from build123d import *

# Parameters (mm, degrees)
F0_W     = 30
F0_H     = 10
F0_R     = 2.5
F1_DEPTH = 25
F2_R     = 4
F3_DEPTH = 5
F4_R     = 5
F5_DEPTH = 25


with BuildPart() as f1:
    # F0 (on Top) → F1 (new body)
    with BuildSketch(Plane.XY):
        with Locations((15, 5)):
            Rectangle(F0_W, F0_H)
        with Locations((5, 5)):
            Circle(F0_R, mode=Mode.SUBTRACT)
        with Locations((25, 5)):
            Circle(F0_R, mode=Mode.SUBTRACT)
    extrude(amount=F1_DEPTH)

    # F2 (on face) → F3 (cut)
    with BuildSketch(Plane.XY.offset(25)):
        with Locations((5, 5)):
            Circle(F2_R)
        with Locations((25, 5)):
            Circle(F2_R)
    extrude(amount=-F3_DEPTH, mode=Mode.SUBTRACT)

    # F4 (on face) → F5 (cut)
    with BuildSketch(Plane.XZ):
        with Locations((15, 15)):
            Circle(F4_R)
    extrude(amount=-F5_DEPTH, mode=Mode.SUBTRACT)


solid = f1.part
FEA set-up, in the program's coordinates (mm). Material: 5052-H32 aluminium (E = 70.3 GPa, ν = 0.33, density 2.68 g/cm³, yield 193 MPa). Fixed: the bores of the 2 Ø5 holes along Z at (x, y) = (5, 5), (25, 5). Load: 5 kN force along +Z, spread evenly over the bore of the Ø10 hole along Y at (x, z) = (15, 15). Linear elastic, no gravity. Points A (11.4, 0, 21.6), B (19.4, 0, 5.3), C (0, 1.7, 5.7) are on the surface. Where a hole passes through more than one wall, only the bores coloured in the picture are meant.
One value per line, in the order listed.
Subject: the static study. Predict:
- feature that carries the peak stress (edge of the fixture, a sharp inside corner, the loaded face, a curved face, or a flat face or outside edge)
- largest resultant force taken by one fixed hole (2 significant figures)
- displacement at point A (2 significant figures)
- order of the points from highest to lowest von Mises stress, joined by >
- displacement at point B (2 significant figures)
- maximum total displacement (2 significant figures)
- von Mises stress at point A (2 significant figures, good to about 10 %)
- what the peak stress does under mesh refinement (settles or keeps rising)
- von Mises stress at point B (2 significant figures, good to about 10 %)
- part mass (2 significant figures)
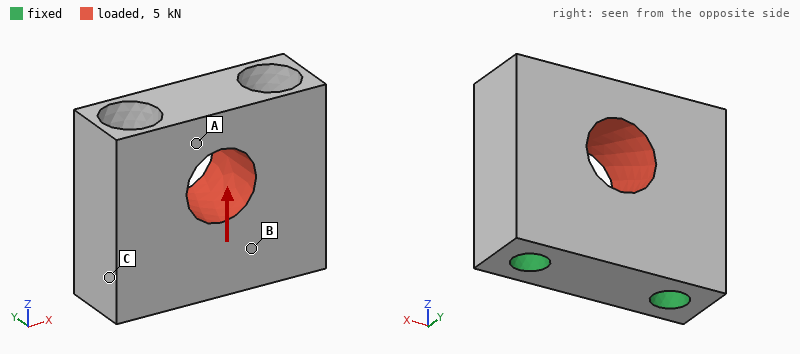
edge of the fixture
2.6 kN
4.0 µm
A > B > C
1.3 µm
5.6 µm
23 MPa
keeps rising
13 MPa
15 g
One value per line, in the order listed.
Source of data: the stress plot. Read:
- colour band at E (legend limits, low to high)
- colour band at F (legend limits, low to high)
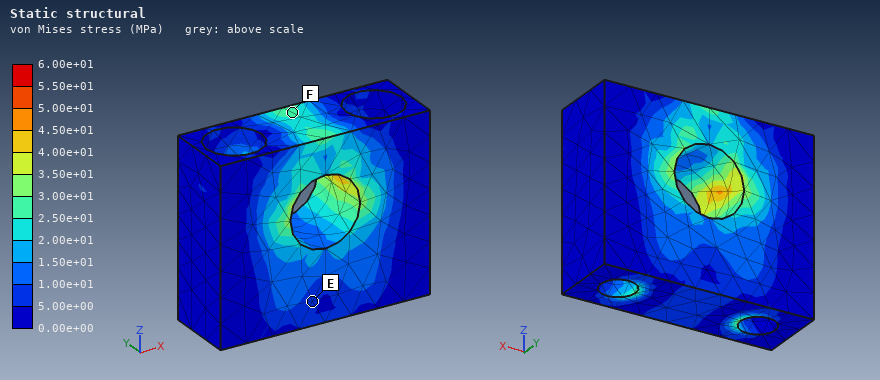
5.00e+00 to 1.00e+01 MPa
2.50e+01 to 3.00e+01 MPa
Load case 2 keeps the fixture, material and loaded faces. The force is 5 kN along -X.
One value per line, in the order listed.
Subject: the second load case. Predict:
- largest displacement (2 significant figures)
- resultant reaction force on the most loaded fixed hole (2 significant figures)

3.2 µm
2.5 kN
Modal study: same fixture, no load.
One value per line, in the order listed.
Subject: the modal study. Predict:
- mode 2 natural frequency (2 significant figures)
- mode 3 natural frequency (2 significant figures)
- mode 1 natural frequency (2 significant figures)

73 kHz
74 kHz
45 kHz
